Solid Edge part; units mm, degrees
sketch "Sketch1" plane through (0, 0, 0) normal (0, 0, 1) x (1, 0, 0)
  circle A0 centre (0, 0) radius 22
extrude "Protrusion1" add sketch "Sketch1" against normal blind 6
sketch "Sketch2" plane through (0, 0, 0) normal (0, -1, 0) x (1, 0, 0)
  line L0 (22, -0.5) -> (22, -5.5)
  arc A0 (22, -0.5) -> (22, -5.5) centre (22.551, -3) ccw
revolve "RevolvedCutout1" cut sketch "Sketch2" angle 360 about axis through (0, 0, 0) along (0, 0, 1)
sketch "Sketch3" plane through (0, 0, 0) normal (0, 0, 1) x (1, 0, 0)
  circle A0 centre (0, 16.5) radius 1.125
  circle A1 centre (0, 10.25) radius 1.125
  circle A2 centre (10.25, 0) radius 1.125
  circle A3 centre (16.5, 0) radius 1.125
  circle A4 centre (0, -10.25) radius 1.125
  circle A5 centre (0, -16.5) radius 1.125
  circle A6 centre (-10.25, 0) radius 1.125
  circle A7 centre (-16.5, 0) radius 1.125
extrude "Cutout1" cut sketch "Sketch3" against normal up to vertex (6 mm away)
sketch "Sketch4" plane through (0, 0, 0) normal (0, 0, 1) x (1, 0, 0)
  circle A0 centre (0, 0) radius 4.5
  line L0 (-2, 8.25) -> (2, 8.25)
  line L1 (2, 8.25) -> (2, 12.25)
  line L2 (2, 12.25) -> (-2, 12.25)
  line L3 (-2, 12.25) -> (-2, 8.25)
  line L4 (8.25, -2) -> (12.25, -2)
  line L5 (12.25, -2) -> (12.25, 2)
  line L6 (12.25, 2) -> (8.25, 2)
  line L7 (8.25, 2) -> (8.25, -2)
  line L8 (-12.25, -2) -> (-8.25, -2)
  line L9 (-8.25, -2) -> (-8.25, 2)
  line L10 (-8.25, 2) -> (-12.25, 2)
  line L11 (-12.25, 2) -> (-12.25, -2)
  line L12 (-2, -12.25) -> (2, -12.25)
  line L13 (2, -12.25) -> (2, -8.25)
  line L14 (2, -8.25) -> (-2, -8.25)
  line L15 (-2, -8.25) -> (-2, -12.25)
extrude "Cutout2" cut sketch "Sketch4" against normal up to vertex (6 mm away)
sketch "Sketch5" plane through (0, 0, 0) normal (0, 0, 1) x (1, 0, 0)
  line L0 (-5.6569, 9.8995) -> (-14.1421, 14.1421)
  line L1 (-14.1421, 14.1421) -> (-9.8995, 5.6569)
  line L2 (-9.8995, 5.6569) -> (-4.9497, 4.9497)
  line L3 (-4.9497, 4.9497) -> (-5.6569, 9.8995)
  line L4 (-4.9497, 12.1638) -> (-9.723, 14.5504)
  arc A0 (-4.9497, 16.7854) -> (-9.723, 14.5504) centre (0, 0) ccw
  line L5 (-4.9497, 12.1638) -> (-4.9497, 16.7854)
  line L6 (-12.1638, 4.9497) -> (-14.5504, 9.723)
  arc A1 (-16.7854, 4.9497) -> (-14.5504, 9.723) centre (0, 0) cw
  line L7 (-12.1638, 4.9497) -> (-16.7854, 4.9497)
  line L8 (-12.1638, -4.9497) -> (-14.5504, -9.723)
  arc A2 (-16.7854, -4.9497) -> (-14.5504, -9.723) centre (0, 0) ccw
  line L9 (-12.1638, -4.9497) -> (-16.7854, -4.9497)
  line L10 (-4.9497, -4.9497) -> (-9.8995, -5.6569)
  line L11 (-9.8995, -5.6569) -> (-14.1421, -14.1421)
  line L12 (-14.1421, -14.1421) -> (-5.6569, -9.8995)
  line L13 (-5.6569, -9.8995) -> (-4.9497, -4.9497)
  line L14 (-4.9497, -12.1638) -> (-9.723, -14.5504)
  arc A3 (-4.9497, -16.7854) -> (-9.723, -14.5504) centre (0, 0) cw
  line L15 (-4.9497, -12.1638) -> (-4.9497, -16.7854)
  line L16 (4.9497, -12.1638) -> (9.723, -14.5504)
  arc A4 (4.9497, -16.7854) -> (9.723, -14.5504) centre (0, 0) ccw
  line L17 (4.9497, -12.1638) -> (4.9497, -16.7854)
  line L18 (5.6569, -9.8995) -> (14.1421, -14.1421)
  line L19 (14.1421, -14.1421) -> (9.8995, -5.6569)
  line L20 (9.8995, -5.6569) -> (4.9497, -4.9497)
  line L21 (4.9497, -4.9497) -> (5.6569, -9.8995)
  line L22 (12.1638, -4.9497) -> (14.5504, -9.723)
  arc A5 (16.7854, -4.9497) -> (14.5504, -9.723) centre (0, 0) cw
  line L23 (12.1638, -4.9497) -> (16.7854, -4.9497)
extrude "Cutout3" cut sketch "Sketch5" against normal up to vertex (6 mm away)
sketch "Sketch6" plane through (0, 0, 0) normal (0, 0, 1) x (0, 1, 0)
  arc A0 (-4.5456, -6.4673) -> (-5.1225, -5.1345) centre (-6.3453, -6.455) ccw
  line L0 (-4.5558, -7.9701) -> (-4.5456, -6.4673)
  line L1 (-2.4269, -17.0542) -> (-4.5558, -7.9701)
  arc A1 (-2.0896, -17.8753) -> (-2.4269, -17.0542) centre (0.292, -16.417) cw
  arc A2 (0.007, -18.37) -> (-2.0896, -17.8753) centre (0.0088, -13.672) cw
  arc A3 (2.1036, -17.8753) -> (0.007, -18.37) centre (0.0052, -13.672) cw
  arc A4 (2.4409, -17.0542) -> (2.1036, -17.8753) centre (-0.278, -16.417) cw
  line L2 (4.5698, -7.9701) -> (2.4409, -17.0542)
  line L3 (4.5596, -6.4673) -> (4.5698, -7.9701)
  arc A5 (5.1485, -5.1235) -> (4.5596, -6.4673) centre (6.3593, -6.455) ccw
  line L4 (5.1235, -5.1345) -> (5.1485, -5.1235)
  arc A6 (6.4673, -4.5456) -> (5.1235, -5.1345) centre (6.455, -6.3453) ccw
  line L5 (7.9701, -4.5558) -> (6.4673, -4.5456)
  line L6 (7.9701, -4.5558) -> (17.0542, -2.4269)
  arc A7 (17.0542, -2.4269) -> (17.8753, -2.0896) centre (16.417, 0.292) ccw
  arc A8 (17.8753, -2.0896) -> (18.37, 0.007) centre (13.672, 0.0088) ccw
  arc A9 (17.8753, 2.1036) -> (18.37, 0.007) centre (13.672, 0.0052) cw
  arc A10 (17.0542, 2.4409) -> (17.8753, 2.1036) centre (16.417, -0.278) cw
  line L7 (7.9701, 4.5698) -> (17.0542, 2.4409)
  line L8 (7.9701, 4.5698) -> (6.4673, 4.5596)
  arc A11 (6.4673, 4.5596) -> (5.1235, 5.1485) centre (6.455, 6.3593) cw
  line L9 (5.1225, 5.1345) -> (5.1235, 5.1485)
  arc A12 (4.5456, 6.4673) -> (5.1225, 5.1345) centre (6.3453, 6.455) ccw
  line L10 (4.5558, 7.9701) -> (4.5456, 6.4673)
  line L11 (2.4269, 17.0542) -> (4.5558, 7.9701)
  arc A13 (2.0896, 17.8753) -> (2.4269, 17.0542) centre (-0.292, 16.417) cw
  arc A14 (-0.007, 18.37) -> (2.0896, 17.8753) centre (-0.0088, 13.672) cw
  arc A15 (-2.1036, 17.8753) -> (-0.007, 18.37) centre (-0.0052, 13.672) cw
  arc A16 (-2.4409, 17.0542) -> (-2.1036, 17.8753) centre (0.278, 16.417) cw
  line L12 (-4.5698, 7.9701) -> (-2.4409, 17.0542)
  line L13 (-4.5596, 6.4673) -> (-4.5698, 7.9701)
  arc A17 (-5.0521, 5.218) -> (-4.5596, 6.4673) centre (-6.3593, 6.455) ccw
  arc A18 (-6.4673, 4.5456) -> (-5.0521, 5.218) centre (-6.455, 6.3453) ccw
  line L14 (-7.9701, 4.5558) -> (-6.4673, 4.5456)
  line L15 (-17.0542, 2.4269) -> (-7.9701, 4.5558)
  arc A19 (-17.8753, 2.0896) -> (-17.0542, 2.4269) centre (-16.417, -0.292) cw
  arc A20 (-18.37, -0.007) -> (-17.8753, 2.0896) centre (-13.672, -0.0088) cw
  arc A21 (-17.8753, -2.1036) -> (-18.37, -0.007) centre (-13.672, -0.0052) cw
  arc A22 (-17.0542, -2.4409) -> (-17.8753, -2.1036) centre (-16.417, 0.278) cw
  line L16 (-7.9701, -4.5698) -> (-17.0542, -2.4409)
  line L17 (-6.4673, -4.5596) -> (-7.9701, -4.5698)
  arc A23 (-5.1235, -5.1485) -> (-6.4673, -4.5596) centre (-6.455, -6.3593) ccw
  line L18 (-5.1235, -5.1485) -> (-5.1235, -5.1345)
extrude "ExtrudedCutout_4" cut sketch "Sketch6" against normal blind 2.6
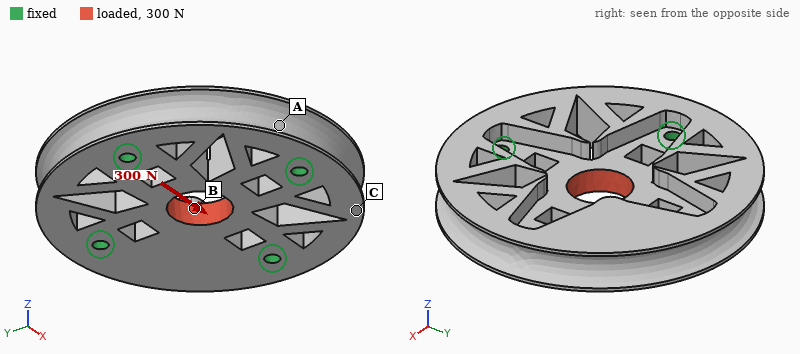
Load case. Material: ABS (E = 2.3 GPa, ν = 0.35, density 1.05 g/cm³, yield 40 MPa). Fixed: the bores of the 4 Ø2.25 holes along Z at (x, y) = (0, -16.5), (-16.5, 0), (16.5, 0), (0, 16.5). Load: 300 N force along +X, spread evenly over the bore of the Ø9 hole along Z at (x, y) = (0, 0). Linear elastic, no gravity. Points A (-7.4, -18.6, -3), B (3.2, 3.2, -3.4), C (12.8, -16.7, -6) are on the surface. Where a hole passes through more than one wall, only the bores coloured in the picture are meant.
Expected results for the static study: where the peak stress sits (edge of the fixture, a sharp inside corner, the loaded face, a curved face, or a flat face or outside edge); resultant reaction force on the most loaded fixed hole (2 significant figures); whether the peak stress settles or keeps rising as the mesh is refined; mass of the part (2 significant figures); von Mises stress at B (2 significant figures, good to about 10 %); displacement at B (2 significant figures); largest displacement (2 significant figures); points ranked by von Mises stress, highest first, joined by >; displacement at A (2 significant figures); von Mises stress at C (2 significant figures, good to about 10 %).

a sharp inside corner
99 N
keeps rising
5.5 g
4.4 MPa
26 µm
32 µm
B > C > A
4.9 µm
1.9 MPa
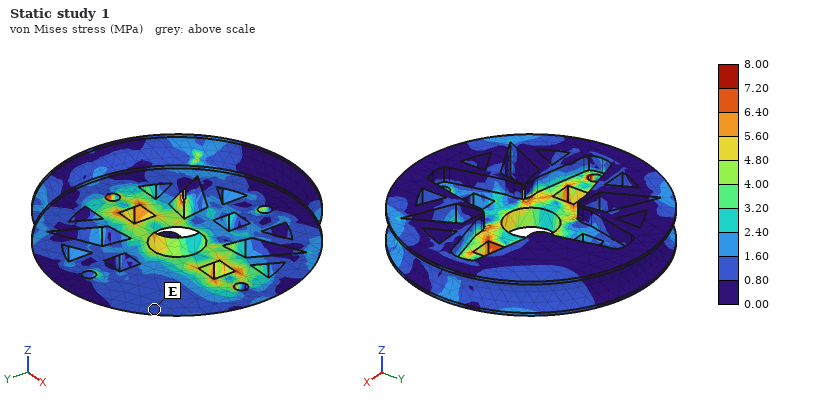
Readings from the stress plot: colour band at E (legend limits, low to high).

0.80 to 1.60 MPa
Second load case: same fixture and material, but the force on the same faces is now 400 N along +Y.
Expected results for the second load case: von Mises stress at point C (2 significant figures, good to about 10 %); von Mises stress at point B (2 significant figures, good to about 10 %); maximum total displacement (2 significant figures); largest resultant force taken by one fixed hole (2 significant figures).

2.1 MPa
6.0 MPa
43 µm
130 N
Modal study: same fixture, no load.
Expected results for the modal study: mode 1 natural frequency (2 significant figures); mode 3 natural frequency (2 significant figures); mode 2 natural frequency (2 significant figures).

5100 Hz
6000 Hz
6000 Hz
